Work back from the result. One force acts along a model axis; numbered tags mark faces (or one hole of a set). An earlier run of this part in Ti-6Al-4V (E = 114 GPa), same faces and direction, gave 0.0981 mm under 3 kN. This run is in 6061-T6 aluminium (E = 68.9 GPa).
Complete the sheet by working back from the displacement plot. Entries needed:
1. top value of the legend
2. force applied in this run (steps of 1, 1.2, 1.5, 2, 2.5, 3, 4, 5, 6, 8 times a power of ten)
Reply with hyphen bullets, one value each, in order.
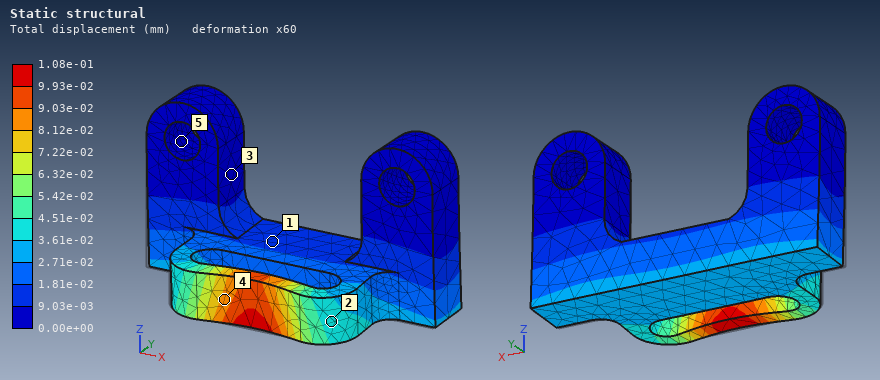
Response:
- 1.08e-01 mm
- 2 kN
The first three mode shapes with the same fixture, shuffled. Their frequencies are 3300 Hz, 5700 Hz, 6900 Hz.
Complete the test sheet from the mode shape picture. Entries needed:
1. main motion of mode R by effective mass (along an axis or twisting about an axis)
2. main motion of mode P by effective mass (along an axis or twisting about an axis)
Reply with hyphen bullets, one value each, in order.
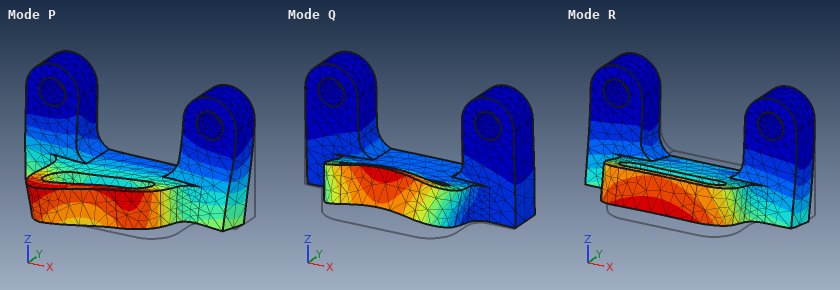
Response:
- along Y
- along X
